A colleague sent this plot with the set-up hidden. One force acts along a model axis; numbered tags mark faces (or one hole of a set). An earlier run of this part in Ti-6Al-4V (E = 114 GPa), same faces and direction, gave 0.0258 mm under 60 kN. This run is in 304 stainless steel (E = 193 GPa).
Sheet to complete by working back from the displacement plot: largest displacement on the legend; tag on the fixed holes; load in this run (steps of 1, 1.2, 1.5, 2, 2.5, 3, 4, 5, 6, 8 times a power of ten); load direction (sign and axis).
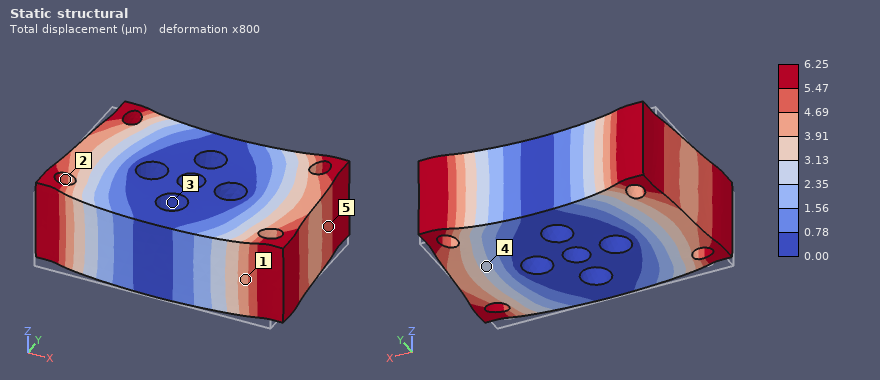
6.25 µm
3
25 kN
+Y
